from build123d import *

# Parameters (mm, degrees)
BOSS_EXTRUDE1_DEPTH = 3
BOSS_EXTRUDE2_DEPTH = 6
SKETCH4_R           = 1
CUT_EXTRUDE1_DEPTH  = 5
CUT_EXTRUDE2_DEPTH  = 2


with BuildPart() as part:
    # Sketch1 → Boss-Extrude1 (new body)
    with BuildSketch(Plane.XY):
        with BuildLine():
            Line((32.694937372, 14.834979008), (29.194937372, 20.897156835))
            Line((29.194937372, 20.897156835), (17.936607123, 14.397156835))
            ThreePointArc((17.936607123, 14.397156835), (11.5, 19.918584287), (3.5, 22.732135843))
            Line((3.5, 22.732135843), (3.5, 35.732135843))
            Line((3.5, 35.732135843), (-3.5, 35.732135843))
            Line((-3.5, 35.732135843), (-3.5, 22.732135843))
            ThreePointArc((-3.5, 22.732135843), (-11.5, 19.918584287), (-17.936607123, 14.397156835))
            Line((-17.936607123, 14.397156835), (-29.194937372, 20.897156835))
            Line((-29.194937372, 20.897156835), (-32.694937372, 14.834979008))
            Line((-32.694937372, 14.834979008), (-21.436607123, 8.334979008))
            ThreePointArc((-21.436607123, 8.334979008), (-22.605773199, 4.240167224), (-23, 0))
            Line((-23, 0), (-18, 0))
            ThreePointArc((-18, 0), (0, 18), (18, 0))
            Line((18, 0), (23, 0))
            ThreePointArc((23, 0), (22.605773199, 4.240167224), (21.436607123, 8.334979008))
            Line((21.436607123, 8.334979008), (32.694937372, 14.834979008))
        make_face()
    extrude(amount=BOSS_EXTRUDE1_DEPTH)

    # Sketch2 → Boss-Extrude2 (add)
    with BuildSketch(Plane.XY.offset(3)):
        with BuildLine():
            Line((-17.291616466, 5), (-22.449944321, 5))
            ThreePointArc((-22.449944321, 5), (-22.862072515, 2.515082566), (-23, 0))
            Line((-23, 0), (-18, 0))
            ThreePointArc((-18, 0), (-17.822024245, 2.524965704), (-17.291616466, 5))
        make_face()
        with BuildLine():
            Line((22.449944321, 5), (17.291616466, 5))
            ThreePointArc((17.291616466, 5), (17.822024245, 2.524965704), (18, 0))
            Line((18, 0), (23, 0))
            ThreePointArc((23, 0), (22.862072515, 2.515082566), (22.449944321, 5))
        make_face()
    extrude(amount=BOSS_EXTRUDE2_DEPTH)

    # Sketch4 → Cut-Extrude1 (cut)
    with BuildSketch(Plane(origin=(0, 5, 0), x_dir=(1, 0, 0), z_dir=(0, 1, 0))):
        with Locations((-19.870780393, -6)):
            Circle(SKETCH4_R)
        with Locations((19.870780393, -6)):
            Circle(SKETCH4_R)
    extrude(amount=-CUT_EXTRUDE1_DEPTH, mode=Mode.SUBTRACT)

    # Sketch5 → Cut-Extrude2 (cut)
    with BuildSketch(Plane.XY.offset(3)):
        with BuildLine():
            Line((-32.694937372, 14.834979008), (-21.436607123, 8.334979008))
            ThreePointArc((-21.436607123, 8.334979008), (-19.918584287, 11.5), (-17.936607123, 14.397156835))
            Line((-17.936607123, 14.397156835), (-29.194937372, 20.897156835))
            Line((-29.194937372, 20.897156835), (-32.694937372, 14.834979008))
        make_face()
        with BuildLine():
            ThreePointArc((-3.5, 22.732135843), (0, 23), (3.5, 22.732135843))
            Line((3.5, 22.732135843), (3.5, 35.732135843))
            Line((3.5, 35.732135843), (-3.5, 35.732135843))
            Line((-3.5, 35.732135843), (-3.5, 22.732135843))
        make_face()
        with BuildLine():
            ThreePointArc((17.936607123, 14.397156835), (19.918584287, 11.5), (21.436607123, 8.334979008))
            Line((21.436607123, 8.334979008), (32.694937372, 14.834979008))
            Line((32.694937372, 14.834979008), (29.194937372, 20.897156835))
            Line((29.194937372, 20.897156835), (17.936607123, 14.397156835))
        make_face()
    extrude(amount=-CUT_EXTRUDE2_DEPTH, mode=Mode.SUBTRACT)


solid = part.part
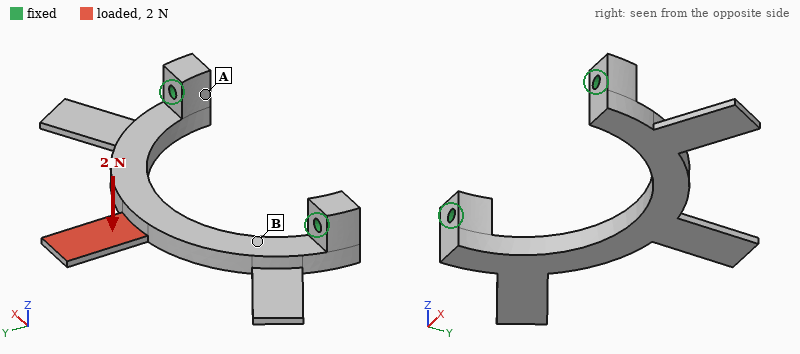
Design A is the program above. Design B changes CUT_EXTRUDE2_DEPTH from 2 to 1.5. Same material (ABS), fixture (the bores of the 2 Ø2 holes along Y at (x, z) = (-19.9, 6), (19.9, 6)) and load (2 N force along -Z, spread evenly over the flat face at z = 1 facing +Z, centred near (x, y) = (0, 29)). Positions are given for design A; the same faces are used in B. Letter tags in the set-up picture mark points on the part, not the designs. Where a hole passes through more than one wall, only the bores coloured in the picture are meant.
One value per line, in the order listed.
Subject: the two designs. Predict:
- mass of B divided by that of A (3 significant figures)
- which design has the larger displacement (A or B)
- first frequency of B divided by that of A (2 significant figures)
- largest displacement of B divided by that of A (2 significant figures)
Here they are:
1.09
A
0.95
0.65
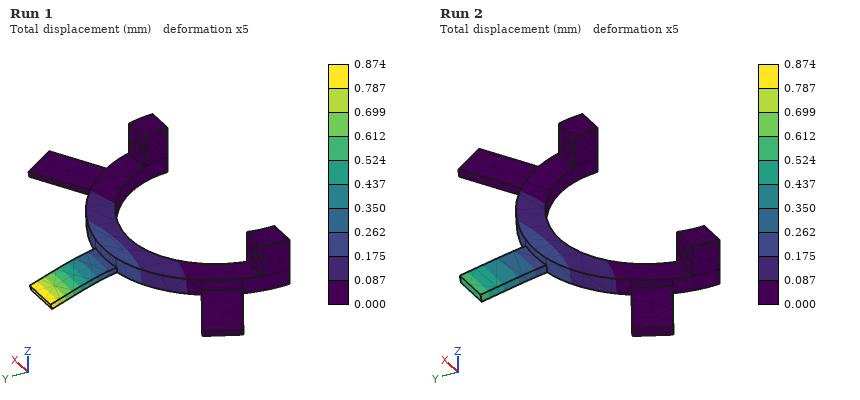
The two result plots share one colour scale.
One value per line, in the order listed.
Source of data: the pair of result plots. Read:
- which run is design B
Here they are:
Run 2
